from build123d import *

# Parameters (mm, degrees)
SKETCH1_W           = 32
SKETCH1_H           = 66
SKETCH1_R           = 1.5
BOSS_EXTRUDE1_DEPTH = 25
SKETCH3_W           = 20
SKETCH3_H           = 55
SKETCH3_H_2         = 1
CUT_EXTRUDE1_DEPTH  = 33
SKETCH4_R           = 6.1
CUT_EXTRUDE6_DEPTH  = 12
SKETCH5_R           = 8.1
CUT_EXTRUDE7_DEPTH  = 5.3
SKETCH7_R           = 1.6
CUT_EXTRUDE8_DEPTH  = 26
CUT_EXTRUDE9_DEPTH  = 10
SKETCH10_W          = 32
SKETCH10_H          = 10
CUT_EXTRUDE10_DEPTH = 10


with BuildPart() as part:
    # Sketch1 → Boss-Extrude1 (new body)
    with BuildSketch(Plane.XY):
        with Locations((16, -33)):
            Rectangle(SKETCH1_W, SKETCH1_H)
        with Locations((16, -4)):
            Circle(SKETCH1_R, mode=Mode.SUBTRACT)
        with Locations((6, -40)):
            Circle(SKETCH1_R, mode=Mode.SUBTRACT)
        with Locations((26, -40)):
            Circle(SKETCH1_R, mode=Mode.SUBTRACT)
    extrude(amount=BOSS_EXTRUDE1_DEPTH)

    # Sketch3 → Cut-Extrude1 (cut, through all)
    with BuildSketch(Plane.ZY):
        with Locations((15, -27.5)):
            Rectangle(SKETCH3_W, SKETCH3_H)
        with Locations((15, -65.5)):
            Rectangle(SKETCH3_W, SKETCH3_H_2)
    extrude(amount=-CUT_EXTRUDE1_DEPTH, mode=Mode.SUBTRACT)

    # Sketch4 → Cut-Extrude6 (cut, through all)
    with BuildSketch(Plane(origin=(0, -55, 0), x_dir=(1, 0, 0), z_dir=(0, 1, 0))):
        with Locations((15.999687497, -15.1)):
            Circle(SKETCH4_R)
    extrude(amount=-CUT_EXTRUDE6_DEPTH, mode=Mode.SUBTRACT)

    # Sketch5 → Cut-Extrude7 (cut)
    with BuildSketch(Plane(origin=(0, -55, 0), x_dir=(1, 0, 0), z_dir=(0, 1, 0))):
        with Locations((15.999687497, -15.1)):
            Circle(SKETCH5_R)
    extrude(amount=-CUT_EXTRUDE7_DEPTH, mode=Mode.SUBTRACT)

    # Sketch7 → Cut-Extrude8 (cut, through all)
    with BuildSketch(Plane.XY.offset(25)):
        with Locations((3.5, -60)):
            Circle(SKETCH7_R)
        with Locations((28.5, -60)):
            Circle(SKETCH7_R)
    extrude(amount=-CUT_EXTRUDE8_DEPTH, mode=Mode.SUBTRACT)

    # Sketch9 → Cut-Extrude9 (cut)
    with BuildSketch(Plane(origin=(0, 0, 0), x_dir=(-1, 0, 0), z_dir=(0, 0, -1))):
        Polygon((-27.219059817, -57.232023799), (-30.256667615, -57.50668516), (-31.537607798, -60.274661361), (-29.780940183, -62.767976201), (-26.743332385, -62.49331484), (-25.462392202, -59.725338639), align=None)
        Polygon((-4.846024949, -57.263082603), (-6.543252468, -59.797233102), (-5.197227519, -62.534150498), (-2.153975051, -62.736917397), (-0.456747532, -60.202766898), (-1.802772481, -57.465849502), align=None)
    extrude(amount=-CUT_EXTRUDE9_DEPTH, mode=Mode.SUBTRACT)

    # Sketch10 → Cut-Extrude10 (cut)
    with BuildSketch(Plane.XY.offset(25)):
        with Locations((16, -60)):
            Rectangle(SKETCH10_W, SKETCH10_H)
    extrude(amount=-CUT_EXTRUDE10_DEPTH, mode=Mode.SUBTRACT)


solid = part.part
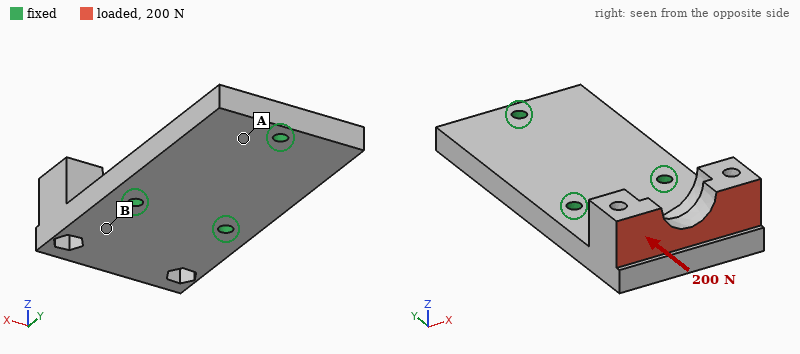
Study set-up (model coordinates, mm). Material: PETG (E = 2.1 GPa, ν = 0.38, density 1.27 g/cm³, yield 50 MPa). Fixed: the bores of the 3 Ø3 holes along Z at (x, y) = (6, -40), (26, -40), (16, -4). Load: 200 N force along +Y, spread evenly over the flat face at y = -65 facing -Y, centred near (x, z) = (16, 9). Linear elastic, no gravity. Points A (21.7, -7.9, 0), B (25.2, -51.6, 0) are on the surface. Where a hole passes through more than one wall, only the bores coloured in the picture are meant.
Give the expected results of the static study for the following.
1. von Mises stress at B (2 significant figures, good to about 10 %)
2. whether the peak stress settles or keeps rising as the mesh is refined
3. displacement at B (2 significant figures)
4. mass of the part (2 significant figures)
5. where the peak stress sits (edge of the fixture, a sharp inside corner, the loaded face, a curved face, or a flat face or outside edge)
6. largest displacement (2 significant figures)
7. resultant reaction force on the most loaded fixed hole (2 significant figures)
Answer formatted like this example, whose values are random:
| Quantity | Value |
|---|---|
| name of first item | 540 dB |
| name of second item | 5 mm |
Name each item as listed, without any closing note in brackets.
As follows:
| Quantity | Value |
|---|---|
| von Mises stress at B | 7.9 MPa |
| whether the peak stress settles or keeps rising as the mesh is refined | keeps rising |
| displacement at B | 0.15 mm |
| mass of the part | 16 g |
| where the peak stress sits | edge of the fixture |
| largest displacement | 0.74 mm |
| resultant reaction force on the most loaded fixed hole | 95 N |
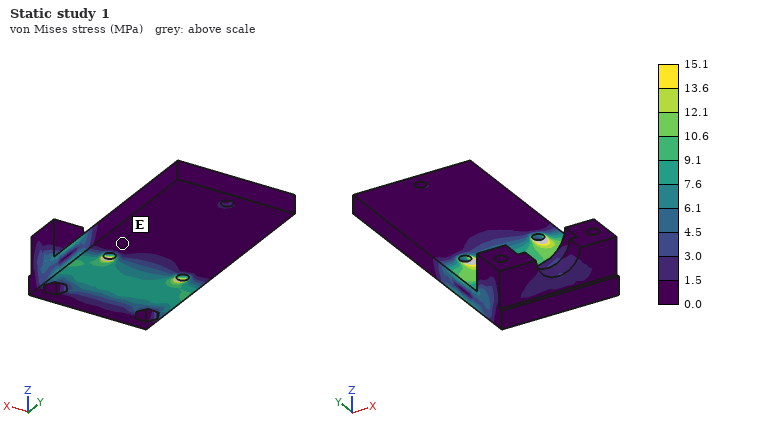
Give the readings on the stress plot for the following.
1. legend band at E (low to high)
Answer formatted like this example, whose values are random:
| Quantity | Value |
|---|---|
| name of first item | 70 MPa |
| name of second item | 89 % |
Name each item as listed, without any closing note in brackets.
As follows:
| Quantity | Value |
|---|---|
| legend band at E | 0.0 to 1.5 MPa |
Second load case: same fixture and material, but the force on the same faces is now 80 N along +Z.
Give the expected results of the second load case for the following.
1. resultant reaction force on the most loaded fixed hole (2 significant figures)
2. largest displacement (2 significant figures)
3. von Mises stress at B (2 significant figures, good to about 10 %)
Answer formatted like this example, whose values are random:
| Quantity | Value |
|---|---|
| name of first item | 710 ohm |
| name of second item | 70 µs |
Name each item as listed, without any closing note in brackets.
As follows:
| Quantity | Value |
|---|---|
| resultant reaction force on the most loaded fixed hole | 45 N |
| largest displacement | 0.75 mm |
| von Mises stress at B | 7.2 MPa |
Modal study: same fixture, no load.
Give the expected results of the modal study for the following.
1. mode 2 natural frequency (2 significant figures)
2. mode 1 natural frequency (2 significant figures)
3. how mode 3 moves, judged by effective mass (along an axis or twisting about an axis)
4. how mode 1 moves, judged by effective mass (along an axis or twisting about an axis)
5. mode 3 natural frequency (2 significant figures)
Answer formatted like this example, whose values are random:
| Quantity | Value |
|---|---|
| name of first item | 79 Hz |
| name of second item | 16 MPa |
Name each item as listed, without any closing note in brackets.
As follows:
| Quantity | Value |
|---|---|
| mode 2 natural frequency | 2100 Hz |
| mode 1 natural frequency | 990 Hz |
| how mode 3 moves, judged by effective mass | twisting about Y |
| how mode 1 moves, judged by effective mass | along Z |
| mode 3 natural frequency | 3200 Hz |
